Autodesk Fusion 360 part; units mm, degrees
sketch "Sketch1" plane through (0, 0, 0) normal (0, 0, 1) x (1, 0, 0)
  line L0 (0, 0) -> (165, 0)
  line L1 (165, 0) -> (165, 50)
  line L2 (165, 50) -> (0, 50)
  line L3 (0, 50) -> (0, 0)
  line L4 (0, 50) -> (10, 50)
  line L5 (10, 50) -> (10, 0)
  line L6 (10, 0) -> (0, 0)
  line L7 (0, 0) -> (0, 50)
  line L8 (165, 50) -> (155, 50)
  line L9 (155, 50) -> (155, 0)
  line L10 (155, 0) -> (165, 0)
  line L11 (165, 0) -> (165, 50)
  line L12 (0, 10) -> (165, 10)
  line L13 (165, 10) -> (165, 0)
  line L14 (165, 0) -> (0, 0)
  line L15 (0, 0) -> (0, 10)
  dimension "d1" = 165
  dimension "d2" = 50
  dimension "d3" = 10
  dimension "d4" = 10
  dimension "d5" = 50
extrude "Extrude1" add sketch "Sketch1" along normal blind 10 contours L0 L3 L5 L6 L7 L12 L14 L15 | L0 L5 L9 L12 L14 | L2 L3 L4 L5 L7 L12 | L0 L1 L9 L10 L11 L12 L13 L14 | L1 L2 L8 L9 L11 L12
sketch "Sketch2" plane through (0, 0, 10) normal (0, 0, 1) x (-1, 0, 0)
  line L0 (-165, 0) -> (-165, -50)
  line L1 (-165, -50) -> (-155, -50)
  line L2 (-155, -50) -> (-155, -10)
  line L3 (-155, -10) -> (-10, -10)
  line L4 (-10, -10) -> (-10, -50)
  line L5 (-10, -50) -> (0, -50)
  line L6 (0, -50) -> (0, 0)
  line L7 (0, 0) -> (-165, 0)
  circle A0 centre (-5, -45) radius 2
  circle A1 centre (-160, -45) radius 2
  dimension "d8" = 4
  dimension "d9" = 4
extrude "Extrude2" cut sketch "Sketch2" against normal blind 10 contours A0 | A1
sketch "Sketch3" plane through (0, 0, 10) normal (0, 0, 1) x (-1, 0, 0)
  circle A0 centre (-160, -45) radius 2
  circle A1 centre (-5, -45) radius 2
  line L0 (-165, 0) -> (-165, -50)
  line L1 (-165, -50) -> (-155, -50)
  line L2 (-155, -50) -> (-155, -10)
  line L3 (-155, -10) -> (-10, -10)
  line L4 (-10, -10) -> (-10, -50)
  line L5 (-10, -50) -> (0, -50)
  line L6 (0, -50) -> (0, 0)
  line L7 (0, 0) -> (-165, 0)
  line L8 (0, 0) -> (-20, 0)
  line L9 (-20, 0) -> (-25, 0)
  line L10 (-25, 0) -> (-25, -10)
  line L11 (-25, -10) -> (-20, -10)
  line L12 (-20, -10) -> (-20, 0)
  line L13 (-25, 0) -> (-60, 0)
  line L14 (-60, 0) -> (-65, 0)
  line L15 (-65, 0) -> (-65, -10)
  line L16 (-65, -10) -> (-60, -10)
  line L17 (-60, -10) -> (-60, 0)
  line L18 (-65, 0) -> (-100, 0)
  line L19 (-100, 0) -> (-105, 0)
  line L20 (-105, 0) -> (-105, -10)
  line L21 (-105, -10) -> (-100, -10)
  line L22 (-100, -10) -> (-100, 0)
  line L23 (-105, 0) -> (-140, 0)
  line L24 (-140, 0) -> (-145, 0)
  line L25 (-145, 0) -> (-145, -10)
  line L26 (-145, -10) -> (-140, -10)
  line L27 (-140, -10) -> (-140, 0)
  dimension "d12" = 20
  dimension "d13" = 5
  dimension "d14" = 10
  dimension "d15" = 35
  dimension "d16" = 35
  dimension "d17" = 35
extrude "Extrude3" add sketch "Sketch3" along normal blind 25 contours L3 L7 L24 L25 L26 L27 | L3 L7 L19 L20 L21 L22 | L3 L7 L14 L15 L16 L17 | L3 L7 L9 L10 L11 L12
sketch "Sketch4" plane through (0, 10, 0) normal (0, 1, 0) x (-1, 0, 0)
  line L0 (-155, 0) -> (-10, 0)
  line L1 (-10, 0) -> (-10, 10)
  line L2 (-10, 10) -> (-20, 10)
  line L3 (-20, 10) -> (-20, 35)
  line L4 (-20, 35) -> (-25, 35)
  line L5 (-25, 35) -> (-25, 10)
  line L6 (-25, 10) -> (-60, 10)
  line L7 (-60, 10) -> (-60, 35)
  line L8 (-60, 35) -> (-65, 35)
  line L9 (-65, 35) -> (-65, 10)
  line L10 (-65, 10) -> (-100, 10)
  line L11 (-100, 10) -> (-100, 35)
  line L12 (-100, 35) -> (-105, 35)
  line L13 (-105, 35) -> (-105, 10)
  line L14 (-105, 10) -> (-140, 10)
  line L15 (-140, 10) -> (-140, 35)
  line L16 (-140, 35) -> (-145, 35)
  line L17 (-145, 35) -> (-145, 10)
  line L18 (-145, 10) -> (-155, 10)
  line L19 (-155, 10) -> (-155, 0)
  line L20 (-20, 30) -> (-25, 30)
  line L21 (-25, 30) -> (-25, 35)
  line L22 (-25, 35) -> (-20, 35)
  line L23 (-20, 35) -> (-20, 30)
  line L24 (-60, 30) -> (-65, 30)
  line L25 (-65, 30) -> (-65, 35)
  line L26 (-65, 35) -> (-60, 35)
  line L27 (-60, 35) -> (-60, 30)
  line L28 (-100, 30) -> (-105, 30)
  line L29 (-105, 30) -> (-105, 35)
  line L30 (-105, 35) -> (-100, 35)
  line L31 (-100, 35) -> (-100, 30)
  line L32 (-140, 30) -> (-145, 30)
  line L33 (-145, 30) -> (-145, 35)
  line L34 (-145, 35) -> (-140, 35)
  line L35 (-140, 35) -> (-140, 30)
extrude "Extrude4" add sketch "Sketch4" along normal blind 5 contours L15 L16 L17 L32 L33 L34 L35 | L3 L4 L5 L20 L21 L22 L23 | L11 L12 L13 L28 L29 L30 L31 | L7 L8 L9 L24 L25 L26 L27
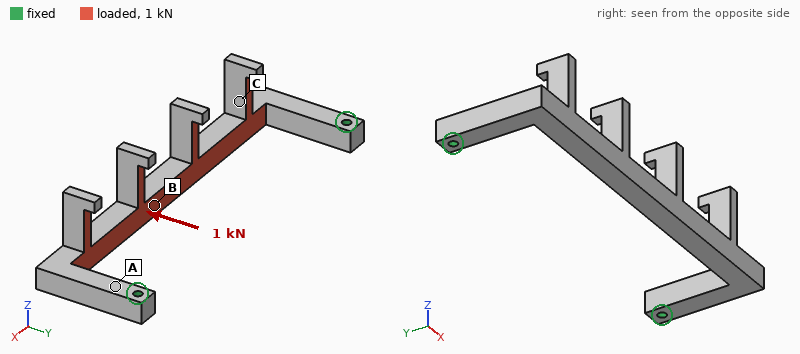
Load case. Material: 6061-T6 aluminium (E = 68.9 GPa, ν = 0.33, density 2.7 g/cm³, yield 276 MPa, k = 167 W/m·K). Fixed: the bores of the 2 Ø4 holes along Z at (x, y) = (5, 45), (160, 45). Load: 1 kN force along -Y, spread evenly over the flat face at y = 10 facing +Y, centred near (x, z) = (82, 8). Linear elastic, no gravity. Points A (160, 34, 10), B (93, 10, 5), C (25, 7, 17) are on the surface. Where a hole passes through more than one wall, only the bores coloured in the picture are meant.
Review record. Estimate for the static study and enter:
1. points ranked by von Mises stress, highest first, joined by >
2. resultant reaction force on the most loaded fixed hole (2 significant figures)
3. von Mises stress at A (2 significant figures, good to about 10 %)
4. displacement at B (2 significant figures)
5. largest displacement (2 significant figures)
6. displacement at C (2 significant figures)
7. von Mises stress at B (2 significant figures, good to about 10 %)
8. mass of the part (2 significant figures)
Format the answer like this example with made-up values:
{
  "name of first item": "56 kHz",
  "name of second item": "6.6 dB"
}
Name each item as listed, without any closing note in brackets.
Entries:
{
  "points ranked by von Mises stress, highest first, joined by >": "B > A > C",
  "resultant reaction force on the most loaded fixed hole": "650 N",
  "von Mises stress at A": "19 MPa",
  "displacement at B": "0.24 mm",
  "largest displacement": "0.32 mm",
  "displacement at C": "0.092 mm",
  "von Mises stress at B": "42 MPa",
  "mass of the part": "80 g"
}
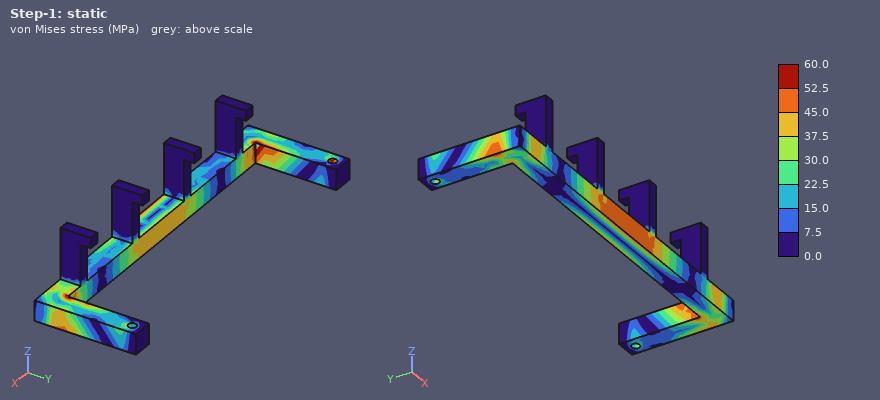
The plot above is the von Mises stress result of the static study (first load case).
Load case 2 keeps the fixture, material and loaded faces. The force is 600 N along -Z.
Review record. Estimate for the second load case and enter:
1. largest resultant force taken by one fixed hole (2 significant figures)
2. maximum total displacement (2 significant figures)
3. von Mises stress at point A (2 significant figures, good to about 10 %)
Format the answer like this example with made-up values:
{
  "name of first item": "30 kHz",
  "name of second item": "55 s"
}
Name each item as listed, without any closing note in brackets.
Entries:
{
  "largest resultant force taken by one fixed hole": "300 N",
  "maximum total displacement": "0.38 mm",
  "von Mises stress at point A": "59 MPa"
}
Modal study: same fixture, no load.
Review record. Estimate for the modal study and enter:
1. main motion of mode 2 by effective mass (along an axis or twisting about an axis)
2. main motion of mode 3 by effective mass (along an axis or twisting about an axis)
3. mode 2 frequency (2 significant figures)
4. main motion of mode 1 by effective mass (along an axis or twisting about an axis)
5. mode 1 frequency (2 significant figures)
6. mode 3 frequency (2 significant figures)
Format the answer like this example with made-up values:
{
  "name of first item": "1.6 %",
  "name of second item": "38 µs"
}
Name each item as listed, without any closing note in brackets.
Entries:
{
  "main motion of mode 2 by effective mass": "along Y",
  "main motion of mode 3 by effective mass": "along X",
  "mode 2 frequency": "1500 Hz",
  "main motion of mode 1 by effective mass": "along Z",
  "mode 1 frequency": "920 Hz",
  "mode 3 frequency": "1700 Hz"
}
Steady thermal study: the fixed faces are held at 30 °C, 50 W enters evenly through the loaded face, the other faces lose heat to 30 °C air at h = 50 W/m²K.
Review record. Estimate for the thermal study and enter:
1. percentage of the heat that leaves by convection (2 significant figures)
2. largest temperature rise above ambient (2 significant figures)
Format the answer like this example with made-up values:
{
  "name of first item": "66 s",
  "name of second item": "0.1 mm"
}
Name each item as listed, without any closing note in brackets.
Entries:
{
  "percentage of the heat that leaves by convection": "45 %",
  "largest temperature rise above ambient": "64 K"
}
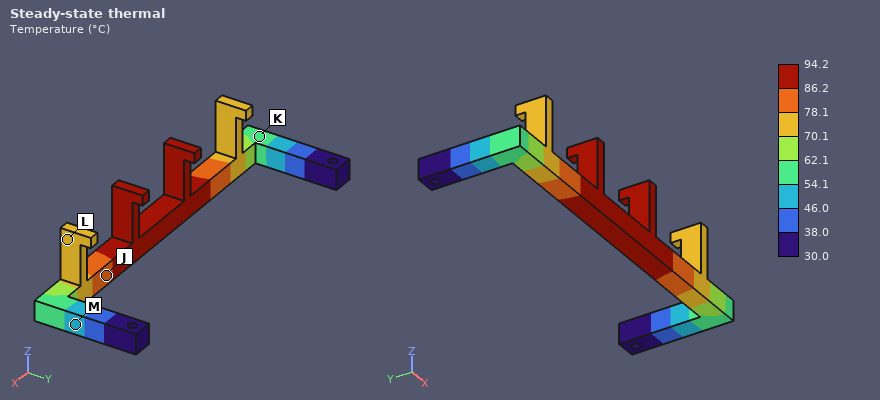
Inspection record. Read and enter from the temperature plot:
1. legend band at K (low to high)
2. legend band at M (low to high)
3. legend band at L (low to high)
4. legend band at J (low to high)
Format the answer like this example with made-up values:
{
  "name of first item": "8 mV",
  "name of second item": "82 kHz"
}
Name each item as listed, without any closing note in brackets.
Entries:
{
  "legend band at K": "54.1 to 62.1 °C",
  "legend band at M": "46.0 to 54.1 °C",
  "legend band at L": "70.1 to 78.1 °C",
  "legend band at J": "78.1 to 86.2 °C"
}
